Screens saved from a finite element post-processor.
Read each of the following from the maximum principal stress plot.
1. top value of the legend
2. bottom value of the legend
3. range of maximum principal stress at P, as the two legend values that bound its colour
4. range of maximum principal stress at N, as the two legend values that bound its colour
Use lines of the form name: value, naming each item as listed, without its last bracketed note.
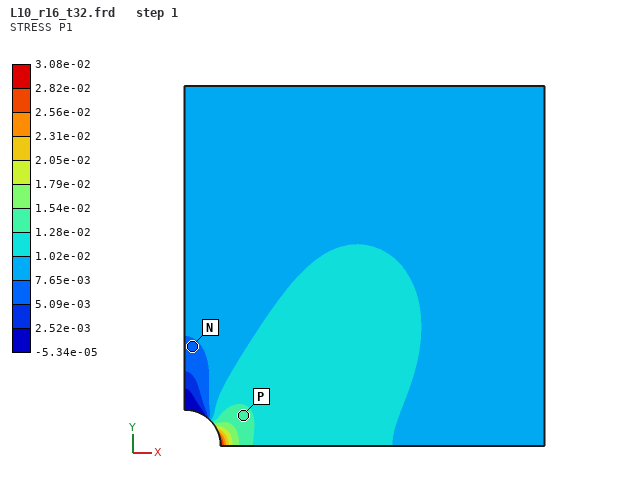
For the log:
top value of the legend: 3.08e-02
bottom value of the legend: -5.34e-05
range of maximum principal stress at P, as the two legend values that bound its colour: 1.28e-02 to 1.54e-02
range of maximum principal stress at N, as the two legend values that bound its colour: 5.09e-03 to 7.65e-03
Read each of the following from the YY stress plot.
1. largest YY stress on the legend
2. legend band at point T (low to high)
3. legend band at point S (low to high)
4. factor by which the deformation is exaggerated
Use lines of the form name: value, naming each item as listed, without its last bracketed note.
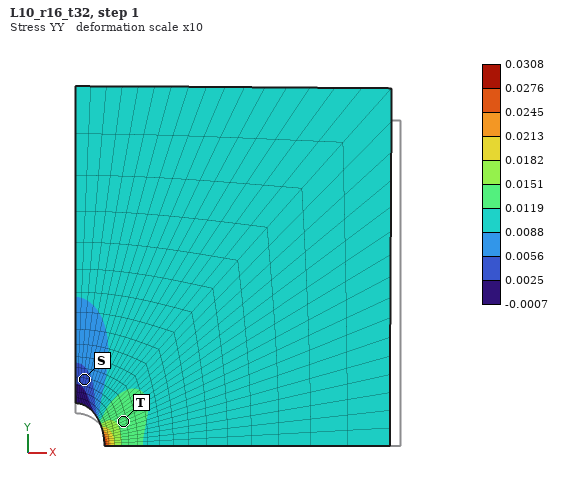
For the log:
largest YY stress on the legend: 0.0308
legend band at point T: 0.0119 to 0.0151
legend band at point S: 0.0025 to 0.0056
factor by which the deformation is exaggerated: 10
